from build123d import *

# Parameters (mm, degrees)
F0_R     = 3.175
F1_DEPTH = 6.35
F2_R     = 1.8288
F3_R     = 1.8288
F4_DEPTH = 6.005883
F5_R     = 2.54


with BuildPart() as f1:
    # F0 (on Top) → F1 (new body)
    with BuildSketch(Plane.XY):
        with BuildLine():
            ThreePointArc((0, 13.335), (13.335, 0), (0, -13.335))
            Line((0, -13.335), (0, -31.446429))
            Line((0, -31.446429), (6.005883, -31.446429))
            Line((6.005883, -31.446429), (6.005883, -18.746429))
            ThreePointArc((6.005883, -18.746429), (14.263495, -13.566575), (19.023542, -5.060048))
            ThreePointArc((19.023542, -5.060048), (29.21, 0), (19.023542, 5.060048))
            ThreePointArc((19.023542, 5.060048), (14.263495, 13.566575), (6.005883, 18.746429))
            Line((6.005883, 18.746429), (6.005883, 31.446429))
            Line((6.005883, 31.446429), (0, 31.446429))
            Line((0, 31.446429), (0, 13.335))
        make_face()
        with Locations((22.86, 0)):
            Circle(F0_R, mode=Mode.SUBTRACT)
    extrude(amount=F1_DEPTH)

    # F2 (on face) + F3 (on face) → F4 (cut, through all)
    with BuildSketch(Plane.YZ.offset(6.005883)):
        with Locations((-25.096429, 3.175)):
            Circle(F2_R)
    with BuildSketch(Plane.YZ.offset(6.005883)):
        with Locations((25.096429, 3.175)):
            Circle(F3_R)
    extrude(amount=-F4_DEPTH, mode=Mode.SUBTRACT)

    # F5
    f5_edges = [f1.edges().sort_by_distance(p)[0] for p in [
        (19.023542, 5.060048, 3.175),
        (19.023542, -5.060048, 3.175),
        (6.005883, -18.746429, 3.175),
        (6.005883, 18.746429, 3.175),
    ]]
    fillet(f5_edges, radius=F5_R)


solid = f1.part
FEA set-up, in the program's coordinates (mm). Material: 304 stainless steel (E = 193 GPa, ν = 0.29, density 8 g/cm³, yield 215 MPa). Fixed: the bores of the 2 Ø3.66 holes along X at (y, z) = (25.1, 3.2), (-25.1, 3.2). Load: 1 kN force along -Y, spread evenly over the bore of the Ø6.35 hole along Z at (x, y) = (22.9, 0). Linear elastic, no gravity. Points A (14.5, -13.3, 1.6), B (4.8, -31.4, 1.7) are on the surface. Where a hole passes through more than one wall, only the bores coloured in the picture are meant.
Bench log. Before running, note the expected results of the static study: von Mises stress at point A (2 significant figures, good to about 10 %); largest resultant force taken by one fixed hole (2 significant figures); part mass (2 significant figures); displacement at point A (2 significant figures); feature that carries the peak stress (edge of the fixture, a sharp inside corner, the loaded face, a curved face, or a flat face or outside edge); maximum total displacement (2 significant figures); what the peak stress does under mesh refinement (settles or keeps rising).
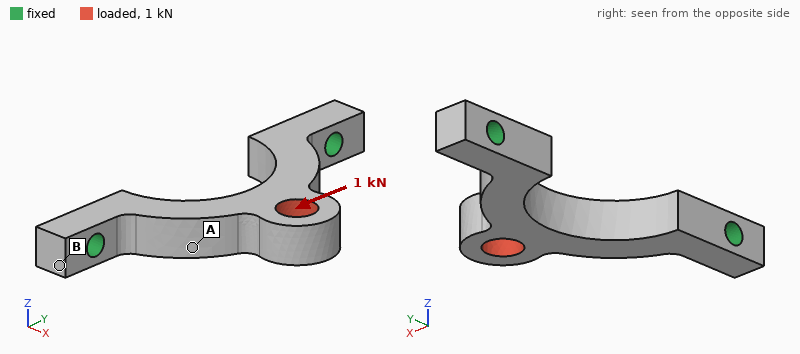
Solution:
16 MPa
690 N
27 g
2.8 µm
edge of the fixture
10.0 µm
keeps rising
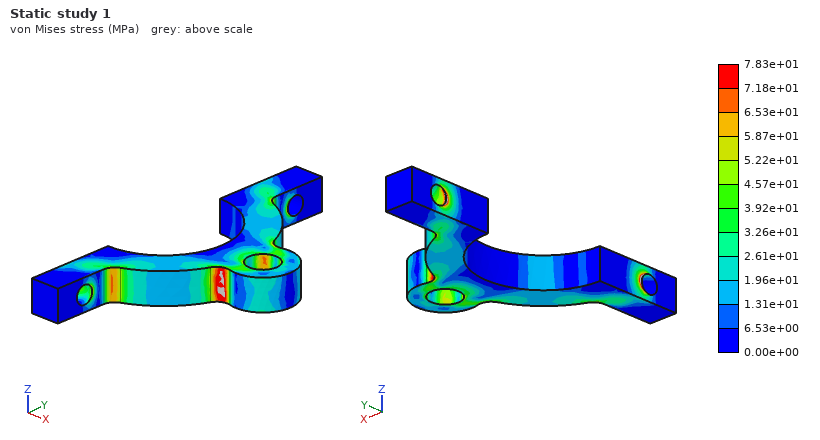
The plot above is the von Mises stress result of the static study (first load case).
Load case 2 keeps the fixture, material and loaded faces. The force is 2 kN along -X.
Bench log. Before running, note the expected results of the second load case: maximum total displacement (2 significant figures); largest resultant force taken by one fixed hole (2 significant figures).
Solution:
12 µm
1.4 kN
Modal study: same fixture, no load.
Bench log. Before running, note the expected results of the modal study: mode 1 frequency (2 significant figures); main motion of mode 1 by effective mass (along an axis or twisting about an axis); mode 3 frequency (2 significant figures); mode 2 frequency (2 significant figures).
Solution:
4400 Hz
along Z
18 kHz
18 kHz
